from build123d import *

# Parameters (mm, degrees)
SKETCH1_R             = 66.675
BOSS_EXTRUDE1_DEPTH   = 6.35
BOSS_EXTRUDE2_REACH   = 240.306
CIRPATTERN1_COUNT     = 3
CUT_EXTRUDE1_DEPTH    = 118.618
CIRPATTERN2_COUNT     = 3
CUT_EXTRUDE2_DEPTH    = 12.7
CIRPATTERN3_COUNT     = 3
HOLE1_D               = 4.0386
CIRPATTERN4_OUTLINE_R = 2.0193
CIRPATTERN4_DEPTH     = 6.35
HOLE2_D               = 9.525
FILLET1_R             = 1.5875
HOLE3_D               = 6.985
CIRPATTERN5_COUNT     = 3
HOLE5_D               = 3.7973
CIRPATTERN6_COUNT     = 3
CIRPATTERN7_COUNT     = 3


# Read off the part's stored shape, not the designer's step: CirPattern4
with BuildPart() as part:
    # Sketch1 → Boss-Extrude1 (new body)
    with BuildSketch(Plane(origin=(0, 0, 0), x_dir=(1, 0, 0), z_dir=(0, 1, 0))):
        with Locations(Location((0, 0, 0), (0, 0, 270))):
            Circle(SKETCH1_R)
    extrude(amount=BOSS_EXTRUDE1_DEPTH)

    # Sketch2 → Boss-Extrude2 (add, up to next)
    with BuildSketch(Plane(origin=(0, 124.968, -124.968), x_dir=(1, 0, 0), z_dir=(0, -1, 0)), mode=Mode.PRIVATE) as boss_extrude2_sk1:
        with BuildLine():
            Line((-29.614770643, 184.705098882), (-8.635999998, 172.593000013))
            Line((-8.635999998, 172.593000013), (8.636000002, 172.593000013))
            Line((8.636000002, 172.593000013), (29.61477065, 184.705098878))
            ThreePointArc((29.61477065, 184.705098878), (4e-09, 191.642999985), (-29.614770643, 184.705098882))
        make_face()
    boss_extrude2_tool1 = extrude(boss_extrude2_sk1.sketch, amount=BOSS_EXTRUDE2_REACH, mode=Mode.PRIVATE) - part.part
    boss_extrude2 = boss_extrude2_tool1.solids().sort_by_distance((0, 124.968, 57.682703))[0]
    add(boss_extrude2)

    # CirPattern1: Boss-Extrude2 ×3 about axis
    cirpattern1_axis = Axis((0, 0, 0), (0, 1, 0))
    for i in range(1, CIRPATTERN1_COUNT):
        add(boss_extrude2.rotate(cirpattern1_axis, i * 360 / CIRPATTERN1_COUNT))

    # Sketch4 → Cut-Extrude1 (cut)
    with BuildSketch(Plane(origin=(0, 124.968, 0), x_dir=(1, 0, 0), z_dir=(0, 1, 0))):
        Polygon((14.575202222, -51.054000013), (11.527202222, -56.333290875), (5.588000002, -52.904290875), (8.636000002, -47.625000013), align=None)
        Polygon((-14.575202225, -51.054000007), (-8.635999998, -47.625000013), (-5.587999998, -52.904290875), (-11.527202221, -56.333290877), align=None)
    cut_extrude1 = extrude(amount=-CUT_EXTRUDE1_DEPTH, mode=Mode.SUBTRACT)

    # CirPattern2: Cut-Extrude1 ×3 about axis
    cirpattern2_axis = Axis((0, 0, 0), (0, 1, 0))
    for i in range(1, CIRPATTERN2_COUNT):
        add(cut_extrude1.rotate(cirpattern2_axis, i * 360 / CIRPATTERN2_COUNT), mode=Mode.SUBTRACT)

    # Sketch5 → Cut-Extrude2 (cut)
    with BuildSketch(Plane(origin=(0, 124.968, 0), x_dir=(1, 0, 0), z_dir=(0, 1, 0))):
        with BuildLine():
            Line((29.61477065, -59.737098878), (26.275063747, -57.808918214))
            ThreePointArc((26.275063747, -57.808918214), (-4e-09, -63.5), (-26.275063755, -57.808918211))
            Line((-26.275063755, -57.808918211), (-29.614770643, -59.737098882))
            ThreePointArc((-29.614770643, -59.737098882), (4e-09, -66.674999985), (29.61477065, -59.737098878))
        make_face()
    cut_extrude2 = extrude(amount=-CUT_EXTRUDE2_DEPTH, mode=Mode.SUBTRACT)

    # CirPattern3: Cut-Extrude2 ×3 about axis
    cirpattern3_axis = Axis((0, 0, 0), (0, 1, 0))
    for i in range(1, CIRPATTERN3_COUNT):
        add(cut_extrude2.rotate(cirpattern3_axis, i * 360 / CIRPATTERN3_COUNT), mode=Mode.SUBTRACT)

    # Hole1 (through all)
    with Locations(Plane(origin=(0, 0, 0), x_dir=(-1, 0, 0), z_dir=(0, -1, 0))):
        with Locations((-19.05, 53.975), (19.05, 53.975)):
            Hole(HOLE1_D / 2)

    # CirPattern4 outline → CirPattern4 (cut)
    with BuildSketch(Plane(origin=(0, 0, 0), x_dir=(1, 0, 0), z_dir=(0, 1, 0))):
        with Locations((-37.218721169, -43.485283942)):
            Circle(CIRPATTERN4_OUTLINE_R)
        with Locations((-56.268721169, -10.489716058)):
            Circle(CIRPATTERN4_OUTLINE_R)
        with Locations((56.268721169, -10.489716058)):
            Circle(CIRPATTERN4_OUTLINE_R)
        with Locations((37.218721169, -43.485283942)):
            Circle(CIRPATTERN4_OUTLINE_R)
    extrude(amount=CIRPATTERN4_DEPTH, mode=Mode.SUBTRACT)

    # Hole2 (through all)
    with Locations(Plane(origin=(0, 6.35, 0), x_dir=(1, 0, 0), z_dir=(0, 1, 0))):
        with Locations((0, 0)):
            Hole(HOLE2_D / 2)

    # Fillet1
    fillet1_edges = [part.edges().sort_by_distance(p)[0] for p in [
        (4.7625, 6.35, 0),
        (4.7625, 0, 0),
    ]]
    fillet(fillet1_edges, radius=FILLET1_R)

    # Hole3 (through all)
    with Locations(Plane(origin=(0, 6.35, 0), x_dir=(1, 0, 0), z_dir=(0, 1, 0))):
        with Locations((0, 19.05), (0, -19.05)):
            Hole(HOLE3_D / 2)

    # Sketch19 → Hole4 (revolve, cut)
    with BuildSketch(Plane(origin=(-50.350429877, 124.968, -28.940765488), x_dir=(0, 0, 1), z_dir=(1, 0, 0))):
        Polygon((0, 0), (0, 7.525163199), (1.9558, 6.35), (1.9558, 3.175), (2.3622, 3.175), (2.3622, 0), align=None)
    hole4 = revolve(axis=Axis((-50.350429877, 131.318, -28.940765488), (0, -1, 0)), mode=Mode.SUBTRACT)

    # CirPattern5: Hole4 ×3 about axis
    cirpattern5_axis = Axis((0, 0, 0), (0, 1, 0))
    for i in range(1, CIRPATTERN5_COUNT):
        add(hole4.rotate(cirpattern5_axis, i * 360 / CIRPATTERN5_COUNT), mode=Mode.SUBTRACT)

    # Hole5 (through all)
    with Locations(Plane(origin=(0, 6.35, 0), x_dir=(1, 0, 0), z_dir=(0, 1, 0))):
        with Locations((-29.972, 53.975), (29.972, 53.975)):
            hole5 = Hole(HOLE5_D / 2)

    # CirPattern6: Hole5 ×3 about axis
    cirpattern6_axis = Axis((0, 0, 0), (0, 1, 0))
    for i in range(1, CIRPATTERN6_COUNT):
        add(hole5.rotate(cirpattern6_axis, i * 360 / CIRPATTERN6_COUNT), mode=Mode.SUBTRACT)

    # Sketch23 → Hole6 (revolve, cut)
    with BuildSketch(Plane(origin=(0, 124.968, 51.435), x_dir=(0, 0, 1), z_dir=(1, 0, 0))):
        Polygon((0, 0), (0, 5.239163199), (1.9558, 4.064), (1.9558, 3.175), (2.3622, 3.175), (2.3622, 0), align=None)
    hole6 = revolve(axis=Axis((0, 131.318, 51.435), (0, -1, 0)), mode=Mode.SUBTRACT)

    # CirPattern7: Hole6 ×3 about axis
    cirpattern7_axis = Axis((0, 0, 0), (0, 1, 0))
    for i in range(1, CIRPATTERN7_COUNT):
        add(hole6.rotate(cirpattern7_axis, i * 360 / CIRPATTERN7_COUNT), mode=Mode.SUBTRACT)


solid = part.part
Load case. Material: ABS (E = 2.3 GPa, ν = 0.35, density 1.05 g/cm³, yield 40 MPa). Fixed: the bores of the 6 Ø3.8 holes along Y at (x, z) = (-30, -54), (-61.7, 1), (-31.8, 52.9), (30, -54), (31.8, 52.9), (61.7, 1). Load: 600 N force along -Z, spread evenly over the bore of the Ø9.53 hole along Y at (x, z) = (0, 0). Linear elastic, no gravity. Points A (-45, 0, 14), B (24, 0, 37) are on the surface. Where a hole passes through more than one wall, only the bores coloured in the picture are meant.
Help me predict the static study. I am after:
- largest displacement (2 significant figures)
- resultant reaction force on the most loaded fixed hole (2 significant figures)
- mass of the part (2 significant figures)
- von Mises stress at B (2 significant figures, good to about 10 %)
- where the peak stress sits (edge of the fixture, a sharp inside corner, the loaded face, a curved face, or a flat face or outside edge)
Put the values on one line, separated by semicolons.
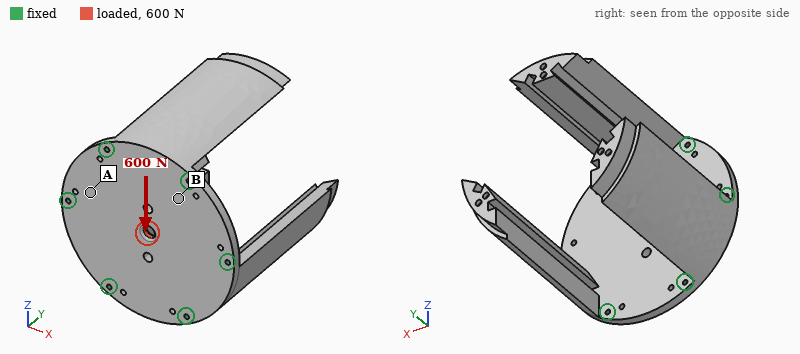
42 µm; 130 N; 330 g; 0.97 MPa; the loaded face
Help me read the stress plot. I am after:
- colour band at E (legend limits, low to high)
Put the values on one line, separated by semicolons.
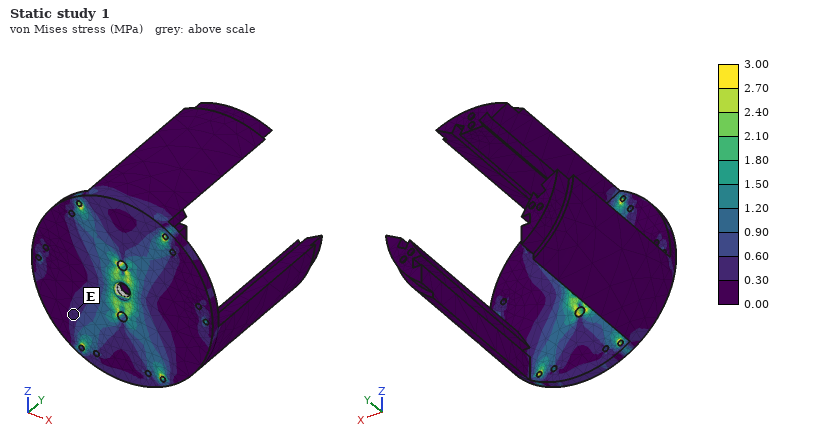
0.30 to 0.60 MPa
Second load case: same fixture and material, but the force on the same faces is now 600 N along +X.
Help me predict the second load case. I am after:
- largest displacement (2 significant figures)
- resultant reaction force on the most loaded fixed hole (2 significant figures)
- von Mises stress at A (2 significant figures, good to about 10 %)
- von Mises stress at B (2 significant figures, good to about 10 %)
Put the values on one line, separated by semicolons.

40 µm; 150 N; 0.53 MPa; 0.58 MPa
